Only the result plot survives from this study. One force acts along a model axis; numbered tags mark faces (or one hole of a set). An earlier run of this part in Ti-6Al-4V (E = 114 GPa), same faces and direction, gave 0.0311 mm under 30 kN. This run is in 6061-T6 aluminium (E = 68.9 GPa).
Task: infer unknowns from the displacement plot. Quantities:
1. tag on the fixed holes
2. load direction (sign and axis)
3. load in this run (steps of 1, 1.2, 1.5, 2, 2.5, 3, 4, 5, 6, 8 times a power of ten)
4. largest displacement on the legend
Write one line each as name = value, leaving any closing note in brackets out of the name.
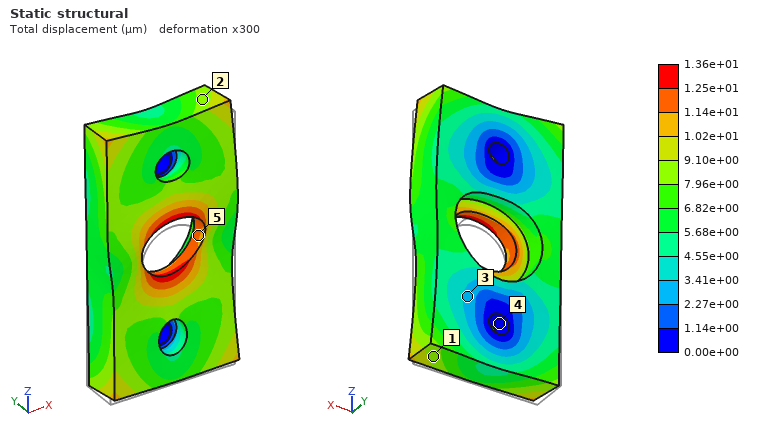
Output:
tag on the fixed holes = 4
load direction = +Z
load in this run = 8 kN
largest displacement on the legend = 1.36e+01 µm
